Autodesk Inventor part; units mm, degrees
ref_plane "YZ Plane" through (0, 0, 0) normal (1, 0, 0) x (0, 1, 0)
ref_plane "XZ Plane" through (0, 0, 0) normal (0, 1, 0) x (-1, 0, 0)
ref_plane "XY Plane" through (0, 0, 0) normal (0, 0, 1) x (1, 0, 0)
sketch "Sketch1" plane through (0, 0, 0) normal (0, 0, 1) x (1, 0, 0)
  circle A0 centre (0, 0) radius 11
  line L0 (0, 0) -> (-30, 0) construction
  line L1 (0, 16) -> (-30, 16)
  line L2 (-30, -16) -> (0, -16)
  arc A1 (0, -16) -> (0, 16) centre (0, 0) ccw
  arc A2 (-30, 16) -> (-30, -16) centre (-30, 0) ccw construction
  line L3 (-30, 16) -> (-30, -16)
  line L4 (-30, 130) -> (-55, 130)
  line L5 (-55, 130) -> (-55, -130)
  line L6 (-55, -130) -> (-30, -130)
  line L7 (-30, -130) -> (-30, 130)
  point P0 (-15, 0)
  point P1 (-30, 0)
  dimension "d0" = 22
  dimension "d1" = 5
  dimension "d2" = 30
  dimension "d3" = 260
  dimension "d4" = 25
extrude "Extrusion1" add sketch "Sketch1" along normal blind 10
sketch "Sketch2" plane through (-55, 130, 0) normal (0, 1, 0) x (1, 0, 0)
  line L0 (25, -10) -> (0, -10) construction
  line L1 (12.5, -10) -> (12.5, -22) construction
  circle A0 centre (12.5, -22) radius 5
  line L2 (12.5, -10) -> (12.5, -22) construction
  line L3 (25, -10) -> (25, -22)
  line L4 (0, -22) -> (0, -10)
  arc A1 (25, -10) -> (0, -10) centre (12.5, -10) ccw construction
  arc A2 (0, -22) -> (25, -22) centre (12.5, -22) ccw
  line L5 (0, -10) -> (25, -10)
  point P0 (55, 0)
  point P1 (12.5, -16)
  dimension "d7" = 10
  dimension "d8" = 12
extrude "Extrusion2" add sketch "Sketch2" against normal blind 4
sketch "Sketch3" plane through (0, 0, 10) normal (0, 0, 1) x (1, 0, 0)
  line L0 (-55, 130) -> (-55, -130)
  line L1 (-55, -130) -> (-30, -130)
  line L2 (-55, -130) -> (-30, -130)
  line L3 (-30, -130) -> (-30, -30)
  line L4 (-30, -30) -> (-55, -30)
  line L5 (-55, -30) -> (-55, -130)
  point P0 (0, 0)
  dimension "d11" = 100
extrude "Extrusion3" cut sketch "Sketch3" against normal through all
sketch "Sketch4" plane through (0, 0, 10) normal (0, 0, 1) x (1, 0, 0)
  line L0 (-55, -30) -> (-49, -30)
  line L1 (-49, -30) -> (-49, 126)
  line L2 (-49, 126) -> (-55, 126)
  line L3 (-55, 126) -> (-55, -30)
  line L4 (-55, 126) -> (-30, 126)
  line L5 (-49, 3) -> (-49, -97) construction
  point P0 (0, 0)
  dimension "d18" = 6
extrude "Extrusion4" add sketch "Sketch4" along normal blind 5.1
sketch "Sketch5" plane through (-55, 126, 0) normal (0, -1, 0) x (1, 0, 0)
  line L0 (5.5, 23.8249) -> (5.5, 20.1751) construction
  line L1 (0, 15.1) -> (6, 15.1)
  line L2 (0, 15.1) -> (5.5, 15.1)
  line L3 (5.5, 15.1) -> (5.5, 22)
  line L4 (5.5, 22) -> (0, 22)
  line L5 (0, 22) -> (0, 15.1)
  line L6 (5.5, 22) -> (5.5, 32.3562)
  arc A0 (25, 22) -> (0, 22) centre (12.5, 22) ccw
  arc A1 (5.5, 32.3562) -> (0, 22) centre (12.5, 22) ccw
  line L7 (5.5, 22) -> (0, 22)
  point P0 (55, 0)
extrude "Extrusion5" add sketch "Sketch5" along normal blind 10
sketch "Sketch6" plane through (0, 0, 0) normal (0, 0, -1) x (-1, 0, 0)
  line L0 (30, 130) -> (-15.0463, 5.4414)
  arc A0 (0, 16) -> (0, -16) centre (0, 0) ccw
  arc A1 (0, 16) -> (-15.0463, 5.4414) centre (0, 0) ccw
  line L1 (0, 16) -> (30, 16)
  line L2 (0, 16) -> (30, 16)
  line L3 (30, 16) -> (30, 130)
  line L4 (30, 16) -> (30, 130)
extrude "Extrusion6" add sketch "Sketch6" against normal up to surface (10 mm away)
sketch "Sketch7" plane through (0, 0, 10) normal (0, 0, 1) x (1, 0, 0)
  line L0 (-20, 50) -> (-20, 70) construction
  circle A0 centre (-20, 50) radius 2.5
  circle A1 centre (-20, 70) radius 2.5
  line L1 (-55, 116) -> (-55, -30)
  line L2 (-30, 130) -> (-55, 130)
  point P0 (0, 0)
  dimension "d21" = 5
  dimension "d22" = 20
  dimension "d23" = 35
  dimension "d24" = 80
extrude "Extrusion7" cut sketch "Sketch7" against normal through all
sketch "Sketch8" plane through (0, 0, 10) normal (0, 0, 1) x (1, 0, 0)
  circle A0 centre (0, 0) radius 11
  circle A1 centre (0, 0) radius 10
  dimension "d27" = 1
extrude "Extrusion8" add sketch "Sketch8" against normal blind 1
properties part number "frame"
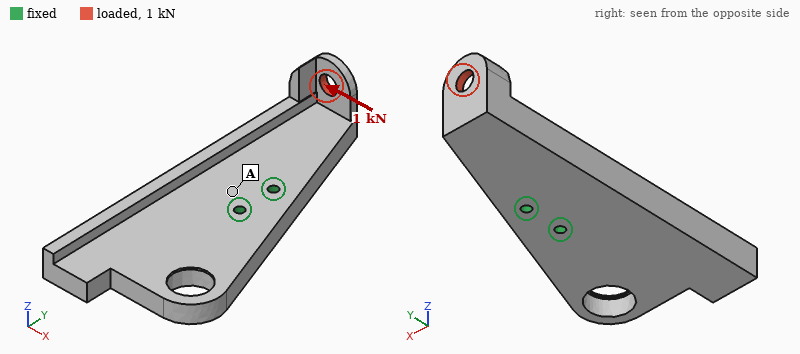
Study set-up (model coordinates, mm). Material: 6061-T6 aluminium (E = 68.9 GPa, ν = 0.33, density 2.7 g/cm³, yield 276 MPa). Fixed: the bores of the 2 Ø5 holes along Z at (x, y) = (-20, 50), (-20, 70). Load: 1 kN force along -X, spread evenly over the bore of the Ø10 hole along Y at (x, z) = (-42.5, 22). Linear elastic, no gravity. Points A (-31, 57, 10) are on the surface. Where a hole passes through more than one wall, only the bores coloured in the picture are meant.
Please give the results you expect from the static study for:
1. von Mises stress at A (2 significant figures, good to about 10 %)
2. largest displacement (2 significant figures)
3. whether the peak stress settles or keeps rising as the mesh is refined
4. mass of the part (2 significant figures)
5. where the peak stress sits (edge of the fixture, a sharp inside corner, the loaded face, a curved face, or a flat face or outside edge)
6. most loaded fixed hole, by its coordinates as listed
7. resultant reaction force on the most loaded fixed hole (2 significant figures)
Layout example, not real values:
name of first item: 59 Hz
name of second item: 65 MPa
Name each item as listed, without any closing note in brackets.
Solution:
von Mises stress at A: 9.3 MPa
largest displacement: 0.20 mm
whether the peak stress settles or keeps rising as the mesh is refined: keeps rising
mass of the part: 220 g
where the peak stress sits: edge of the fixture
most loaded fixed hole, by its coordinates as listed: (-20, 70)
resultant reaction force on the most loaded fixed hole: 3.4 kN
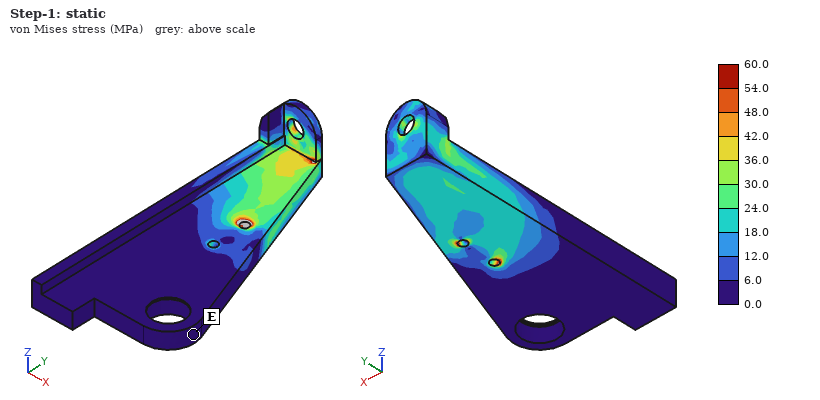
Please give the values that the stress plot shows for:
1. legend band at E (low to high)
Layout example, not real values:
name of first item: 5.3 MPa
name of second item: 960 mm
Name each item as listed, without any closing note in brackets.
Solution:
legend band at E: 0.0 to 6.0 MPa
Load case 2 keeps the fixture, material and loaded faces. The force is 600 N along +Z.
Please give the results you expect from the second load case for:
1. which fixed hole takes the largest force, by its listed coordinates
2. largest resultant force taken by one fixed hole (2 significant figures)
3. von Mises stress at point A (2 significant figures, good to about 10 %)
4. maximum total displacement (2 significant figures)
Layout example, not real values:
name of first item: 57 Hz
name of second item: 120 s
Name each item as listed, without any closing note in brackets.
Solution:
which fixed hole takes the largest force, by its listed coordinates: (-20, 70)
largest resultant force taken by one fixed hole: 1.4 kN
von Mises stress at point A: 17 MPa
maximum total displacement: 0.25 mm
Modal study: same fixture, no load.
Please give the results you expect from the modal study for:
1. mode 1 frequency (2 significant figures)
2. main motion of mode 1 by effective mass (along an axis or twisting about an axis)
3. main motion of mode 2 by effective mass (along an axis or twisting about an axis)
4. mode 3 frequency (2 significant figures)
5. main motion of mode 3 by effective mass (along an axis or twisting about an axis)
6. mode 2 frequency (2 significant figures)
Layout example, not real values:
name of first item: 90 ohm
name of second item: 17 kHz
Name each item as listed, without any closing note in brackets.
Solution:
mode 1 frequency: 1300 Hz
main motion of mode 1 by effective mass: along Z
main motion of mode 2 by effective mass: along Z
mode 3 frequency: 2800 Hz
main motion of mode 3 by effective mass: twisting about Y
mode 2 frequency: 1800 Hz
